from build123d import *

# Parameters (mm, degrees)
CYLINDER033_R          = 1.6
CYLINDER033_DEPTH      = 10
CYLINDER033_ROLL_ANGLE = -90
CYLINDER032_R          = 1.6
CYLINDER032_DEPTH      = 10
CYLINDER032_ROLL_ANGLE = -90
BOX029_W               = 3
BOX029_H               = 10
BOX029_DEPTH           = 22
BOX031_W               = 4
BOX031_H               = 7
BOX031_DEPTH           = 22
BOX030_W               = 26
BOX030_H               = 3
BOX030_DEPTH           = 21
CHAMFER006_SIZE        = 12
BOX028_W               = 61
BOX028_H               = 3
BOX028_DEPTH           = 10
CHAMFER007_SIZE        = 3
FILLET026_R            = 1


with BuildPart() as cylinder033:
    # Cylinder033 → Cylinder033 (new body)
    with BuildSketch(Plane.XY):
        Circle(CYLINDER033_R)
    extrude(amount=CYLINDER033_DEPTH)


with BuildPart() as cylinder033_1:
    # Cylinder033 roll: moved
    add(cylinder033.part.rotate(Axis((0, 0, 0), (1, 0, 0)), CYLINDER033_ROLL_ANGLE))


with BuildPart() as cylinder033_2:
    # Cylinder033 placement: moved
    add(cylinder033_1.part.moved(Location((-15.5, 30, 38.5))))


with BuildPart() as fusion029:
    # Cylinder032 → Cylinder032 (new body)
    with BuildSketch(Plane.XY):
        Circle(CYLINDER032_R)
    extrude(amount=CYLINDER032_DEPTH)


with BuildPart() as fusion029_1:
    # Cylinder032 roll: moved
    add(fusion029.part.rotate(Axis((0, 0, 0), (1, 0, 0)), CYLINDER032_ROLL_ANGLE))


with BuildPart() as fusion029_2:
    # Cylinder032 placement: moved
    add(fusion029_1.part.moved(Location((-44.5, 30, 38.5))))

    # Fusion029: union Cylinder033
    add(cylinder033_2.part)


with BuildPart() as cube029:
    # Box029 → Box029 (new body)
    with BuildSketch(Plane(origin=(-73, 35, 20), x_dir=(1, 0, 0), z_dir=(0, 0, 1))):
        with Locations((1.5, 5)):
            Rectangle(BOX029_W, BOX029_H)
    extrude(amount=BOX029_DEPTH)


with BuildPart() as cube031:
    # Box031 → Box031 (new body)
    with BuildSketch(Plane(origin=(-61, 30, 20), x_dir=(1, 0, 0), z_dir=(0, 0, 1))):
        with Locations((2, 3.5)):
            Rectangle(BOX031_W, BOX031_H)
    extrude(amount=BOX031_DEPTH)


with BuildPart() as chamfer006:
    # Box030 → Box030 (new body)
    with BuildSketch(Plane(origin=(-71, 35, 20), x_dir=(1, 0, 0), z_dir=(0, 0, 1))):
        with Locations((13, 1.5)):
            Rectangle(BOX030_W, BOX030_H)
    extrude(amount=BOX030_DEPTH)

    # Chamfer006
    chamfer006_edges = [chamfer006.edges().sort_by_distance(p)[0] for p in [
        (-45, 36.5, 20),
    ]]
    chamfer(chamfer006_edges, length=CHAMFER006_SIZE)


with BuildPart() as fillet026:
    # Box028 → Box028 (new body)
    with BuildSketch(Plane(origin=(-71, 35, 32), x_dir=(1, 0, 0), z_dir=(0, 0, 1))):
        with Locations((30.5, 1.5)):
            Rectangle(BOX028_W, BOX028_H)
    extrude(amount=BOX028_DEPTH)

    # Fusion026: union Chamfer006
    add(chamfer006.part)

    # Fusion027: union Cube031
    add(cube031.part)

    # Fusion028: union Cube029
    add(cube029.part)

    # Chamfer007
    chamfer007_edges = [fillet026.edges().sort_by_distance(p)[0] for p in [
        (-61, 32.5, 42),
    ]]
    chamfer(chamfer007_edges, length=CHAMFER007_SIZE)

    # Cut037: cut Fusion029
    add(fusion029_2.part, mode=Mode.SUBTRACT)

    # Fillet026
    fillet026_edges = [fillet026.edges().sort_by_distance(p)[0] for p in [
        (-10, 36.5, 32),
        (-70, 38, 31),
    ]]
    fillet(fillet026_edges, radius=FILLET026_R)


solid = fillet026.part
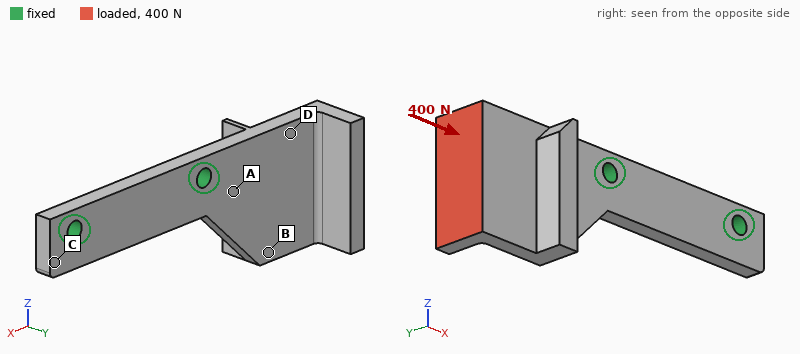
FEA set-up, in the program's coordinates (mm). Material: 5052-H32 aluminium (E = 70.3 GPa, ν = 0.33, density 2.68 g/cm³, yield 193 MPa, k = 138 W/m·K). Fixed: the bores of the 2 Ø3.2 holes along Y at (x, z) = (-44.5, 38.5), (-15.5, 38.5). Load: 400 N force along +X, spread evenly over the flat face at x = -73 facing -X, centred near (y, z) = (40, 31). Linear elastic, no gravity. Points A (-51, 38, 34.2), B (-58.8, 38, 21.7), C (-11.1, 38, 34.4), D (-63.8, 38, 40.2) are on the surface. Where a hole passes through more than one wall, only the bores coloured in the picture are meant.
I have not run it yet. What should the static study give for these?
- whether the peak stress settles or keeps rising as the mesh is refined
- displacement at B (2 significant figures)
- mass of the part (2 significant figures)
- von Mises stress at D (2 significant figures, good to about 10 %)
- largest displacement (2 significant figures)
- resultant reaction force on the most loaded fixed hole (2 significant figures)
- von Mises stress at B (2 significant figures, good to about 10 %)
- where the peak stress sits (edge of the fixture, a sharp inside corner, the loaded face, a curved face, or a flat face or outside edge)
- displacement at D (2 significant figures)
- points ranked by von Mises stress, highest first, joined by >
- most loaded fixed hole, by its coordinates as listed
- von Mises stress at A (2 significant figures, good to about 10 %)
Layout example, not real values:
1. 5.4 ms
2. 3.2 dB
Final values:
1. keeps rising
2. 0.090 mm
3. 9.4 g
4. 47 MPa
5. 0.28 mm
6. 300 N
7. 20 MPa
8. edge of the fixture
9. 0.11 mm
10. A > D > B > C
11. (-44.5, 38.5)
12. 78 MPa
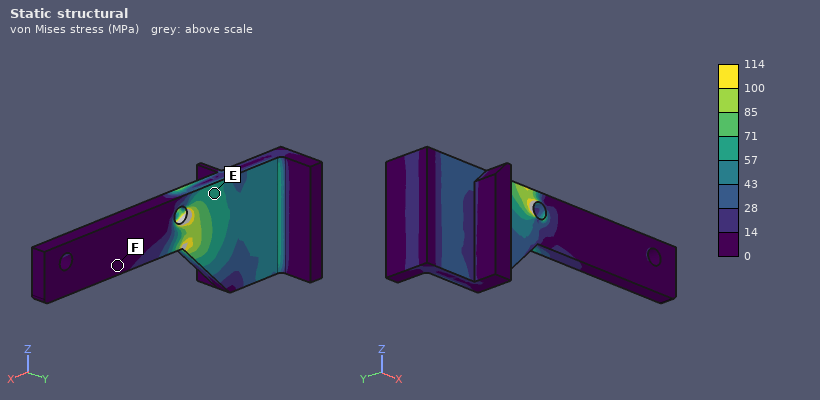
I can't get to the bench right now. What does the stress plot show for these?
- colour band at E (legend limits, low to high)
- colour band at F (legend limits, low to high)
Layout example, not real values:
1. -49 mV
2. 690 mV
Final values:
1. 57 to 71 MPa
2. 0 to 14 MPa
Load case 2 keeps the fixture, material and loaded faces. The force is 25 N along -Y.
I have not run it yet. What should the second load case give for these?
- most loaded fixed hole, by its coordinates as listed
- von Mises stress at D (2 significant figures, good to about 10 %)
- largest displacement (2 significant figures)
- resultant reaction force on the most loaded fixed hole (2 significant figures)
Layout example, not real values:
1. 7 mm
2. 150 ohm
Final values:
1. (-44.5, 38.5)
2. 7.5 MPa
3. 0.11 mm
4. 27 N
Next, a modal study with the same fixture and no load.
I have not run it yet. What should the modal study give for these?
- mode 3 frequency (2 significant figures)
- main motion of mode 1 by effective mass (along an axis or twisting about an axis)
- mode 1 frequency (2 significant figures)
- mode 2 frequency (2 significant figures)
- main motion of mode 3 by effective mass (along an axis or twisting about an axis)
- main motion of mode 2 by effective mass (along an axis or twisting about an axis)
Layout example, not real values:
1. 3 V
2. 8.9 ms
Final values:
1. 4600 Hz
2. along Y
3. 1600 Hz
4. 3900 Hz
5. along Z
6. along Z
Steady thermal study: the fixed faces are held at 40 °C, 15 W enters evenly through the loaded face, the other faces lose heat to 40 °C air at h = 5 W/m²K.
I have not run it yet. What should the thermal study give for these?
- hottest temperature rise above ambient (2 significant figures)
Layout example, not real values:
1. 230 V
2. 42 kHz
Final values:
1. 63 K
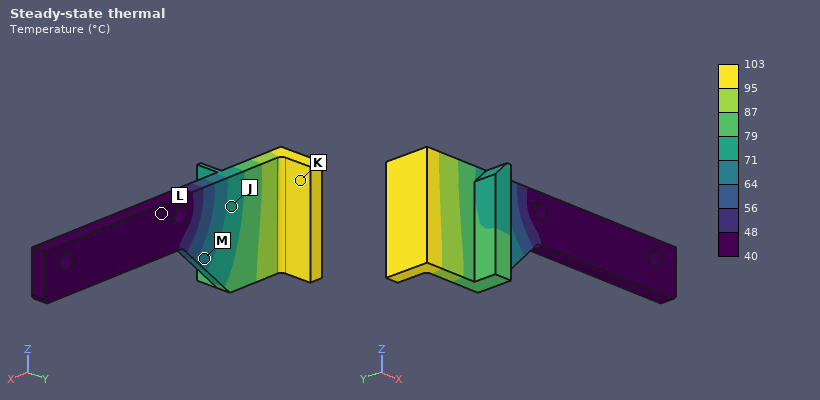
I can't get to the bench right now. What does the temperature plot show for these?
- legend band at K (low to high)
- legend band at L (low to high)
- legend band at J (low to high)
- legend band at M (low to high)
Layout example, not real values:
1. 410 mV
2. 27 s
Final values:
1. 95 to 103 °C
2. 40 to 48 °C
3. 71 to 79 °C
4. 64 to 71 °C
